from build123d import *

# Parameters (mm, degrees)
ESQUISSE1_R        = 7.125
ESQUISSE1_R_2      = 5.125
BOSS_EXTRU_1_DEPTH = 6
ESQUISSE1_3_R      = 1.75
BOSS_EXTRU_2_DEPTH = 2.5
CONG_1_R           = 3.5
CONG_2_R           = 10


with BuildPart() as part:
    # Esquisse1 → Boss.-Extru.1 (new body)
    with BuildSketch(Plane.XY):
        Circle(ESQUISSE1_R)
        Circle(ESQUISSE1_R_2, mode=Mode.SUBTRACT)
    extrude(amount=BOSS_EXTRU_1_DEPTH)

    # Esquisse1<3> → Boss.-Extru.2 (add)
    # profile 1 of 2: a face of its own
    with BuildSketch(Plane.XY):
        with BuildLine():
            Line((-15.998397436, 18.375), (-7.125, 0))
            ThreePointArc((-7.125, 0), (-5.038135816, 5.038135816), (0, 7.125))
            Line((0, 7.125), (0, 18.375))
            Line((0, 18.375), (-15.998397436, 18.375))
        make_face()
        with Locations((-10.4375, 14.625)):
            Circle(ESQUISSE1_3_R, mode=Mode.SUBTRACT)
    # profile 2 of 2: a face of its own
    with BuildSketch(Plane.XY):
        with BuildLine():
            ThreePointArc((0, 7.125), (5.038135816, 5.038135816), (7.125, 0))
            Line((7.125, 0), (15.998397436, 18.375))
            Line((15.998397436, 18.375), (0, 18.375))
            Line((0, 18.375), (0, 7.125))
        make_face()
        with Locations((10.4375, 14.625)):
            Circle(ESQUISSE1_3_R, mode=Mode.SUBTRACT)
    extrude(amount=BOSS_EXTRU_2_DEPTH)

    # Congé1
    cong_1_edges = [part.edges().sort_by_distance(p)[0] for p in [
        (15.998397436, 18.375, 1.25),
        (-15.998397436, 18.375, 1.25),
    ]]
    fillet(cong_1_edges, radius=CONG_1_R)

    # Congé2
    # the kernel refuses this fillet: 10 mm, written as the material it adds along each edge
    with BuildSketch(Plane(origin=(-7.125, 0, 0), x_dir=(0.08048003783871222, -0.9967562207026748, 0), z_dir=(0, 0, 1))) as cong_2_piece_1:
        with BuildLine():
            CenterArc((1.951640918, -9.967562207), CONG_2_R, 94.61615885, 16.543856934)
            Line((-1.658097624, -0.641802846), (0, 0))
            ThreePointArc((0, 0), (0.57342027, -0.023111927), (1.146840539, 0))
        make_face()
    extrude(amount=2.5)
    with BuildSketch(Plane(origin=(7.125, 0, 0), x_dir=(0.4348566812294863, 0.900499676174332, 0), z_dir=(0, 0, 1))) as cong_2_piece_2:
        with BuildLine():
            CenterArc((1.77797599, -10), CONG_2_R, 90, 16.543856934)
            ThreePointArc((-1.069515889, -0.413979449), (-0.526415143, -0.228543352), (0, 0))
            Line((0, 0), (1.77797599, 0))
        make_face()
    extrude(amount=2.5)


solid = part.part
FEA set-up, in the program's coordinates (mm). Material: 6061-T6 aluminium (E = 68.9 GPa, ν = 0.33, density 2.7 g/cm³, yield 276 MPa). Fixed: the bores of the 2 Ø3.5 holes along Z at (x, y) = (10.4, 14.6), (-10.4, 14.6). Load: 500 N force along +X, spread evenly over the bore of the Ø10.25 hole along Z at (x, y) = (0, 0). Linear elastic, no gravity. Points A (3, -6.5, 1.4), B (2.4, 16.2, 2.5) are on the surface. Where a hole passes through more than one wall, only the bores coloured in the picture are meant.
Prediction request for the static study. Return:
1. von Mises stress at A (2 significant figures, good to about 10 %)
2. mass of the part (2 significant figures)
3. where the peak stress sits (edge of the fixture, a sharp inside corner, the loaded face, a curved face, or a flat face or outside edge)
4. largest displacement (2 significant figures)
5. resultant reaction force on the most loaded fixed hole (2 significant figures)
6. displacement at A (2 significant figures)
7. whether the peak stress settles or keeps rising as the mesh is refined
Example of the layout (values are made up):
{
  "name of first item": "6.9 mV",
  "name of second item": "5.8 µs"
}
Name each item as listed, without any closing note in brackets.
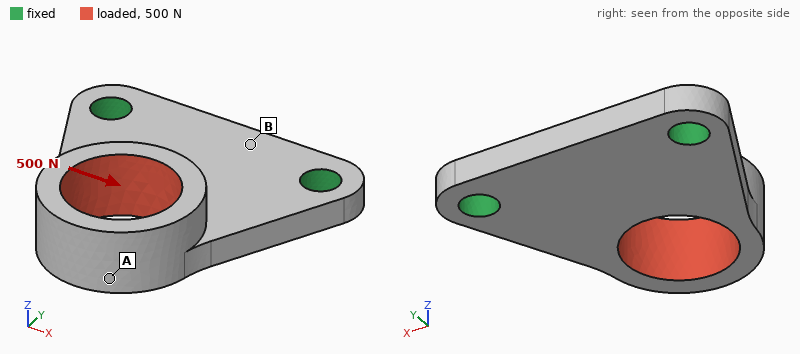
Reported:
{
  "von Mises stress at A": "29 MPa",
  "mass of the part": "3.4 g",
  "where the peak stress sits": "a sharp inside corner",
  "largest displacement": "32 µm",
  "resultant reaction force on the most loaded fixed hole": "420 N",
  "displacement at A": "26 µm",
  "whether the peak stress settles or keeps rising as the mesh is refined": "keeps rising"
}
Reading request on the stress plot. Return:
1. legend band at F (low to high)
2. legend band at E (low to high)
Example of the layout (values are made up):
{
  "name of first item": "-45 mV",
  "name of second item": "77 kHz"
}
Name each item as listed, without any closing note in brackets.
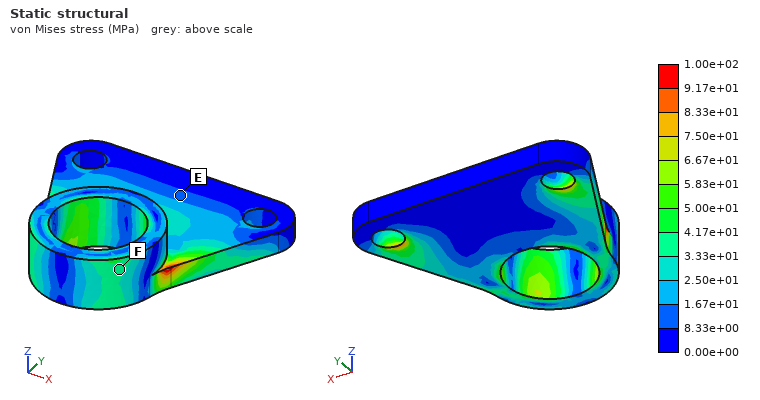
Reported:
{
  "legend band at F": "3.33e+01 to 4.17e+01 MPa",
  "legend band at E": "8.33e+00 to 1.67e+01 MPa"
}
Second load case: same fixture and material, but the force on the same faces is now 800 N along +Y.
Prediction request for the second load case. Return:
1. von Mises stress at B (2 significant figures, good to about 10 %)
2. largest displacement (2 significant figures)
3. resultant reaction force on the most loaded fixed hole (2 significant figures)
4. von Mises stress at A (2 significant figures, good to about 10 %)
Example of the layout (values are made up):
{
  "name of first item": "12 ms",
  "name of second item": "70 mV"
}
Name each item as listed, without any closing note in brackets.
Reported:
{
  "von Mises stress at B": "17 MPa",
  "largest displacement": "0.15 mm",
  "resultant reaction force on the most loaded fixed hole": "430 N",
  "von Mises stress at A": "21 MPa"
}
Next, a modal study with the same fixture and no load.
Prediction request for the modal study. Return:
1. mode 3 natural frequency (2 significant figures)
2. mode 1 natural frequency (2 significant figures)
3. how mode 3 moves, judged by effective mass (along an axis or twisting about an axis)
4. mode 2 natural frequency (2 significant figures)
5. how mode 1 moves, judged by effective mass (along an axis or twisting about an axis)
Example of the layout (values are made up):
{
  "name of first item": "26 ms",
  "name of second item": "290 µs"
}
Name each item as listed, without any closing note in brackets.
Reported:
{
  "mode 3 natural frequency": "22 kHz",
  "mode 1 natural frequency": "5200 Hz",
  "how mode 3 moves, judged by effective mass": "along X",
  "mode 2 natural frequency": "16 kHz",
  "how mode 1 moves, judged by effective mass": "along Z"
}
